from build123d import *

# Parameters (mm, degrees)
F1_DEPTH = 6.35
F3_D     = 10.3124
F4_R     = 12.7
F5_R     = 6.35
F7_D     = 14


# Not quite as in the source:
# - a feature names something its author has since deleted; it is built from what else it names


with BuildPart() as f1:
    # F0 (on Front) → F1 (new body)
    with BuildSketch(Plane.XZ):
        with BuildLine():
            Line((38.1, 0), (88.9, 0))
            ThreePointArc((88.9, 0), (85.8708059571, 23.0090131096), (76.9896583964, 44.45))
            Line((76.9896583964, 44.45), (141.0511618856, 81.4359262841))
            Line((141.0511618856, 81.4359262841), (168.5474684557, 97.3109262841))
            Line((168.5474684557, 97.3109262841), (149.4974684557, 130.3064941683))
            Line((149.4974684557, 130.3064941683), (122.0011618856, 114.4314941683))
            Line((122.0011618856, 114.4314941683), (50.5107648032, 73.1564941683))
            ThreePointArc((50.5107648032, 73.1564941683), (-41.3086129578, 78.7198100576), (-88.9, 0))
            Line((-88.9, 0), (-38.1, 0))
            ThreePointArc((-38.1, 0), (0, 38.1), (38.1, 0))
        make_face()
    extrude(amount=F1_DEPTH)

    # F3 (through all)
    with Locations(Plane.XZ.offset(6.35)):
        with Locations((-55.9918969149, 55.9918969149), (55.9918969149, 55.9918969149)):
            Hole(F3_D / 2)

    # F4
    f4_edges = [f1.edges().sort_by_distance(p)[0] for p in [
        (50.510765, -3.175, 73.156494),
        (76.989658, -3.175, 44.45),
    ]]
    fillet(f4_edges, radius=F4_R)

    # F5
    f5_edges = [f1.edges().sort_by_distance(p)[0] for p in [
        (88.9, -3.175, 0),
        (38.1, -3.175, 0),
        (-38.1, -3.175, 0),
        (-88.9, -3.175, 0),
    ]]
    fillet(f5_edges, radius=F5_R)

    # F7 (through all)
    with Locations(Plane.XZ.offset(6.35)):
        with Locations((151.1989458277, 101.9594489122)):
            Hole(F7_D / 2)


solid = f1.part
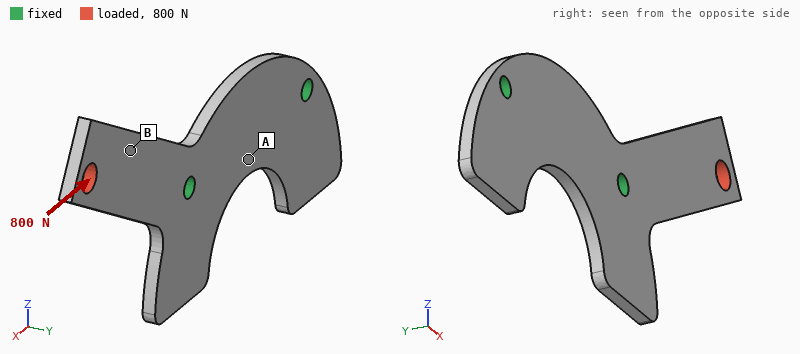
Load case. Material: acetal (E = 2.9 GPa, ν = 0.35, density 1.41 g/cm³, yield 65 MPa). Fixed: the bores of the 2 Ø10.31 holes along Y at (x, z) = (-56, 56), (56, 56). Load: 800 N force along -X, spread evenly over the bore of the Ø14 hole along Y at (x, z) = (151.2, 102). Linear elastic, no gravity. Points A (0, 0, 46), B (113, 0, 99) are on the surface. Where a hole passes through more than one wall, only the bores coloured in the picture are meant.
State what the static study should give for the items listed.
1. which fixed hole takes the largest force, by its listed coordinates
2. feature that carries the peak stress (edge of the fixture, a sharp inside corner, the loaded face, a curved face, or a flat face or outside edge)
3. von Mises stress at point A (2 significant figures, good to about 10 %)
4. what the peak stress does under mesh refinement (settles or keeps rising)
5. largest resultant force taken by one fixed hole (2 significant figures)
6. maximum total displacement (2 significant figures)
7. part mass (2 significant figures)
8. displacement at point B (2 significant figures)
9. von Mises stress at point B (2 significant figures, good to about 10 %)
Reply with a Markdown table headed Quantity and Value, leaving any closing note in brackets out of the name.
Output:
| Quantity | Value |
|---|---|
| which fixed hole takes the largest force, by its listed coordinates | (56, 56) |
| feature that carries the peak stress | edge of the fixture |
| von Mises stress at point A | 2.7 MPa |
| what the peak stress does under mesh refinement | keeps rising |
| largest resultant force taken by one fixed hole | 700 N |
| maximum total displacement | 2.4 mm |
| part mass | 120 g |
| displacement at point B | 1.2 mm |
| von Mises stress at point B | 6.9 MPa |
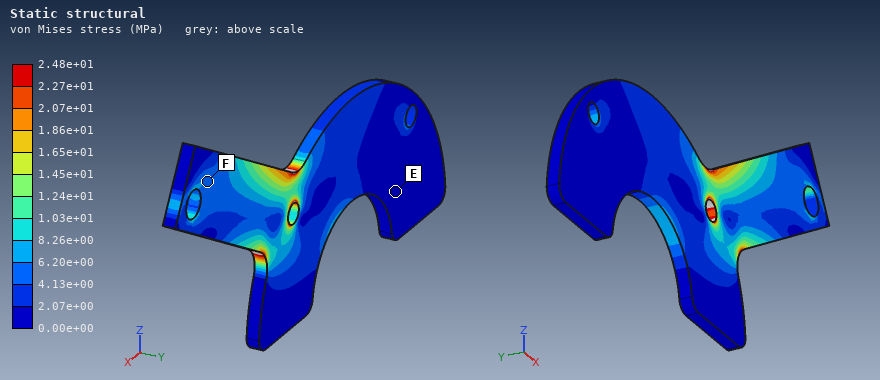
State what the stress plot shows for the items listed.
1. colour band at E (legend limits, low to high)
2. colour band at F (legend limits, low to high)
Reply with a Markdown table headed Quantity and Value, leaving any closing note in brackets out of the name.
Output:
| Quantity | Value |
|---|---|
| colour band at E | 0.00e+00 to 2.07e+00 MPa |
| colour band at F | 4.13e+00 to 6.20e+00 MPa |
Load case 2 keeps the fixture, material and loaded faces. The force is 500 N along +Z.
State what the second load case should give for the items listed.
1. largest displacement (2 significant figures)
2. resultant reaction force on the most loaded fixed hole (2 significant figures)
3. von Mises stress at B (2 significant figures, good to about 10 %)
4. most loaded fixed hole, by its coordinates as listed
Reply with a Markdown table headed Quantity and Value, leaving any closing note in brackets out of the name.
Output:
| Quantity | Value |
|---|---|
| largest displacement | 3.2 mm |
| resultant reaction force on the most loaded fixed hole | 810 N |
| von Mises stress at B | 5.9 MPa |
| most loaded fixed hole, by its coordinates as listed | (56, 56) |
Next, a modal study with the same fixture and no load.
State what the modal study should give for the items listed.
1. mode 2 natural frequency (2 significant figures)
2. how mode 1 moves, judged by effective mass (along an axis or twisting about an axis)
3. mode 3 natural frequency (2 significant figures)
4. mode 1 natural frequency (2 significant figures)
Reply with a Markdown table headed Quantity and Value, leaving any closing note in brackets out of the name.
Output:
| Quantity | Value |
|---|---|
| mode 2 natural frequency | 470 Hz |
| how mode 1 moves, judged by effective mass | along Y |
| mode 3 natural frequency | 510 Hz |
| mode 1 natural frequency | 120 Hz |
